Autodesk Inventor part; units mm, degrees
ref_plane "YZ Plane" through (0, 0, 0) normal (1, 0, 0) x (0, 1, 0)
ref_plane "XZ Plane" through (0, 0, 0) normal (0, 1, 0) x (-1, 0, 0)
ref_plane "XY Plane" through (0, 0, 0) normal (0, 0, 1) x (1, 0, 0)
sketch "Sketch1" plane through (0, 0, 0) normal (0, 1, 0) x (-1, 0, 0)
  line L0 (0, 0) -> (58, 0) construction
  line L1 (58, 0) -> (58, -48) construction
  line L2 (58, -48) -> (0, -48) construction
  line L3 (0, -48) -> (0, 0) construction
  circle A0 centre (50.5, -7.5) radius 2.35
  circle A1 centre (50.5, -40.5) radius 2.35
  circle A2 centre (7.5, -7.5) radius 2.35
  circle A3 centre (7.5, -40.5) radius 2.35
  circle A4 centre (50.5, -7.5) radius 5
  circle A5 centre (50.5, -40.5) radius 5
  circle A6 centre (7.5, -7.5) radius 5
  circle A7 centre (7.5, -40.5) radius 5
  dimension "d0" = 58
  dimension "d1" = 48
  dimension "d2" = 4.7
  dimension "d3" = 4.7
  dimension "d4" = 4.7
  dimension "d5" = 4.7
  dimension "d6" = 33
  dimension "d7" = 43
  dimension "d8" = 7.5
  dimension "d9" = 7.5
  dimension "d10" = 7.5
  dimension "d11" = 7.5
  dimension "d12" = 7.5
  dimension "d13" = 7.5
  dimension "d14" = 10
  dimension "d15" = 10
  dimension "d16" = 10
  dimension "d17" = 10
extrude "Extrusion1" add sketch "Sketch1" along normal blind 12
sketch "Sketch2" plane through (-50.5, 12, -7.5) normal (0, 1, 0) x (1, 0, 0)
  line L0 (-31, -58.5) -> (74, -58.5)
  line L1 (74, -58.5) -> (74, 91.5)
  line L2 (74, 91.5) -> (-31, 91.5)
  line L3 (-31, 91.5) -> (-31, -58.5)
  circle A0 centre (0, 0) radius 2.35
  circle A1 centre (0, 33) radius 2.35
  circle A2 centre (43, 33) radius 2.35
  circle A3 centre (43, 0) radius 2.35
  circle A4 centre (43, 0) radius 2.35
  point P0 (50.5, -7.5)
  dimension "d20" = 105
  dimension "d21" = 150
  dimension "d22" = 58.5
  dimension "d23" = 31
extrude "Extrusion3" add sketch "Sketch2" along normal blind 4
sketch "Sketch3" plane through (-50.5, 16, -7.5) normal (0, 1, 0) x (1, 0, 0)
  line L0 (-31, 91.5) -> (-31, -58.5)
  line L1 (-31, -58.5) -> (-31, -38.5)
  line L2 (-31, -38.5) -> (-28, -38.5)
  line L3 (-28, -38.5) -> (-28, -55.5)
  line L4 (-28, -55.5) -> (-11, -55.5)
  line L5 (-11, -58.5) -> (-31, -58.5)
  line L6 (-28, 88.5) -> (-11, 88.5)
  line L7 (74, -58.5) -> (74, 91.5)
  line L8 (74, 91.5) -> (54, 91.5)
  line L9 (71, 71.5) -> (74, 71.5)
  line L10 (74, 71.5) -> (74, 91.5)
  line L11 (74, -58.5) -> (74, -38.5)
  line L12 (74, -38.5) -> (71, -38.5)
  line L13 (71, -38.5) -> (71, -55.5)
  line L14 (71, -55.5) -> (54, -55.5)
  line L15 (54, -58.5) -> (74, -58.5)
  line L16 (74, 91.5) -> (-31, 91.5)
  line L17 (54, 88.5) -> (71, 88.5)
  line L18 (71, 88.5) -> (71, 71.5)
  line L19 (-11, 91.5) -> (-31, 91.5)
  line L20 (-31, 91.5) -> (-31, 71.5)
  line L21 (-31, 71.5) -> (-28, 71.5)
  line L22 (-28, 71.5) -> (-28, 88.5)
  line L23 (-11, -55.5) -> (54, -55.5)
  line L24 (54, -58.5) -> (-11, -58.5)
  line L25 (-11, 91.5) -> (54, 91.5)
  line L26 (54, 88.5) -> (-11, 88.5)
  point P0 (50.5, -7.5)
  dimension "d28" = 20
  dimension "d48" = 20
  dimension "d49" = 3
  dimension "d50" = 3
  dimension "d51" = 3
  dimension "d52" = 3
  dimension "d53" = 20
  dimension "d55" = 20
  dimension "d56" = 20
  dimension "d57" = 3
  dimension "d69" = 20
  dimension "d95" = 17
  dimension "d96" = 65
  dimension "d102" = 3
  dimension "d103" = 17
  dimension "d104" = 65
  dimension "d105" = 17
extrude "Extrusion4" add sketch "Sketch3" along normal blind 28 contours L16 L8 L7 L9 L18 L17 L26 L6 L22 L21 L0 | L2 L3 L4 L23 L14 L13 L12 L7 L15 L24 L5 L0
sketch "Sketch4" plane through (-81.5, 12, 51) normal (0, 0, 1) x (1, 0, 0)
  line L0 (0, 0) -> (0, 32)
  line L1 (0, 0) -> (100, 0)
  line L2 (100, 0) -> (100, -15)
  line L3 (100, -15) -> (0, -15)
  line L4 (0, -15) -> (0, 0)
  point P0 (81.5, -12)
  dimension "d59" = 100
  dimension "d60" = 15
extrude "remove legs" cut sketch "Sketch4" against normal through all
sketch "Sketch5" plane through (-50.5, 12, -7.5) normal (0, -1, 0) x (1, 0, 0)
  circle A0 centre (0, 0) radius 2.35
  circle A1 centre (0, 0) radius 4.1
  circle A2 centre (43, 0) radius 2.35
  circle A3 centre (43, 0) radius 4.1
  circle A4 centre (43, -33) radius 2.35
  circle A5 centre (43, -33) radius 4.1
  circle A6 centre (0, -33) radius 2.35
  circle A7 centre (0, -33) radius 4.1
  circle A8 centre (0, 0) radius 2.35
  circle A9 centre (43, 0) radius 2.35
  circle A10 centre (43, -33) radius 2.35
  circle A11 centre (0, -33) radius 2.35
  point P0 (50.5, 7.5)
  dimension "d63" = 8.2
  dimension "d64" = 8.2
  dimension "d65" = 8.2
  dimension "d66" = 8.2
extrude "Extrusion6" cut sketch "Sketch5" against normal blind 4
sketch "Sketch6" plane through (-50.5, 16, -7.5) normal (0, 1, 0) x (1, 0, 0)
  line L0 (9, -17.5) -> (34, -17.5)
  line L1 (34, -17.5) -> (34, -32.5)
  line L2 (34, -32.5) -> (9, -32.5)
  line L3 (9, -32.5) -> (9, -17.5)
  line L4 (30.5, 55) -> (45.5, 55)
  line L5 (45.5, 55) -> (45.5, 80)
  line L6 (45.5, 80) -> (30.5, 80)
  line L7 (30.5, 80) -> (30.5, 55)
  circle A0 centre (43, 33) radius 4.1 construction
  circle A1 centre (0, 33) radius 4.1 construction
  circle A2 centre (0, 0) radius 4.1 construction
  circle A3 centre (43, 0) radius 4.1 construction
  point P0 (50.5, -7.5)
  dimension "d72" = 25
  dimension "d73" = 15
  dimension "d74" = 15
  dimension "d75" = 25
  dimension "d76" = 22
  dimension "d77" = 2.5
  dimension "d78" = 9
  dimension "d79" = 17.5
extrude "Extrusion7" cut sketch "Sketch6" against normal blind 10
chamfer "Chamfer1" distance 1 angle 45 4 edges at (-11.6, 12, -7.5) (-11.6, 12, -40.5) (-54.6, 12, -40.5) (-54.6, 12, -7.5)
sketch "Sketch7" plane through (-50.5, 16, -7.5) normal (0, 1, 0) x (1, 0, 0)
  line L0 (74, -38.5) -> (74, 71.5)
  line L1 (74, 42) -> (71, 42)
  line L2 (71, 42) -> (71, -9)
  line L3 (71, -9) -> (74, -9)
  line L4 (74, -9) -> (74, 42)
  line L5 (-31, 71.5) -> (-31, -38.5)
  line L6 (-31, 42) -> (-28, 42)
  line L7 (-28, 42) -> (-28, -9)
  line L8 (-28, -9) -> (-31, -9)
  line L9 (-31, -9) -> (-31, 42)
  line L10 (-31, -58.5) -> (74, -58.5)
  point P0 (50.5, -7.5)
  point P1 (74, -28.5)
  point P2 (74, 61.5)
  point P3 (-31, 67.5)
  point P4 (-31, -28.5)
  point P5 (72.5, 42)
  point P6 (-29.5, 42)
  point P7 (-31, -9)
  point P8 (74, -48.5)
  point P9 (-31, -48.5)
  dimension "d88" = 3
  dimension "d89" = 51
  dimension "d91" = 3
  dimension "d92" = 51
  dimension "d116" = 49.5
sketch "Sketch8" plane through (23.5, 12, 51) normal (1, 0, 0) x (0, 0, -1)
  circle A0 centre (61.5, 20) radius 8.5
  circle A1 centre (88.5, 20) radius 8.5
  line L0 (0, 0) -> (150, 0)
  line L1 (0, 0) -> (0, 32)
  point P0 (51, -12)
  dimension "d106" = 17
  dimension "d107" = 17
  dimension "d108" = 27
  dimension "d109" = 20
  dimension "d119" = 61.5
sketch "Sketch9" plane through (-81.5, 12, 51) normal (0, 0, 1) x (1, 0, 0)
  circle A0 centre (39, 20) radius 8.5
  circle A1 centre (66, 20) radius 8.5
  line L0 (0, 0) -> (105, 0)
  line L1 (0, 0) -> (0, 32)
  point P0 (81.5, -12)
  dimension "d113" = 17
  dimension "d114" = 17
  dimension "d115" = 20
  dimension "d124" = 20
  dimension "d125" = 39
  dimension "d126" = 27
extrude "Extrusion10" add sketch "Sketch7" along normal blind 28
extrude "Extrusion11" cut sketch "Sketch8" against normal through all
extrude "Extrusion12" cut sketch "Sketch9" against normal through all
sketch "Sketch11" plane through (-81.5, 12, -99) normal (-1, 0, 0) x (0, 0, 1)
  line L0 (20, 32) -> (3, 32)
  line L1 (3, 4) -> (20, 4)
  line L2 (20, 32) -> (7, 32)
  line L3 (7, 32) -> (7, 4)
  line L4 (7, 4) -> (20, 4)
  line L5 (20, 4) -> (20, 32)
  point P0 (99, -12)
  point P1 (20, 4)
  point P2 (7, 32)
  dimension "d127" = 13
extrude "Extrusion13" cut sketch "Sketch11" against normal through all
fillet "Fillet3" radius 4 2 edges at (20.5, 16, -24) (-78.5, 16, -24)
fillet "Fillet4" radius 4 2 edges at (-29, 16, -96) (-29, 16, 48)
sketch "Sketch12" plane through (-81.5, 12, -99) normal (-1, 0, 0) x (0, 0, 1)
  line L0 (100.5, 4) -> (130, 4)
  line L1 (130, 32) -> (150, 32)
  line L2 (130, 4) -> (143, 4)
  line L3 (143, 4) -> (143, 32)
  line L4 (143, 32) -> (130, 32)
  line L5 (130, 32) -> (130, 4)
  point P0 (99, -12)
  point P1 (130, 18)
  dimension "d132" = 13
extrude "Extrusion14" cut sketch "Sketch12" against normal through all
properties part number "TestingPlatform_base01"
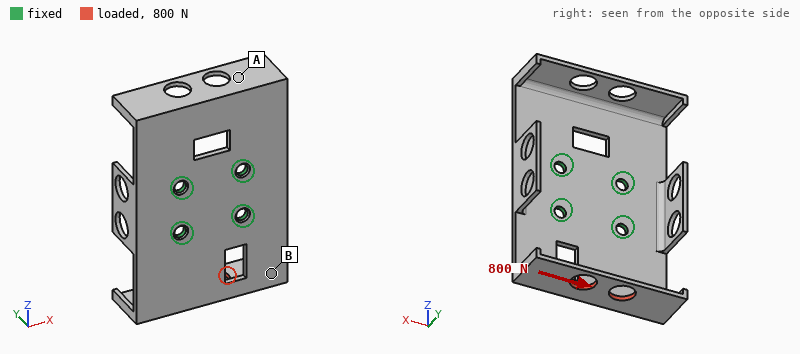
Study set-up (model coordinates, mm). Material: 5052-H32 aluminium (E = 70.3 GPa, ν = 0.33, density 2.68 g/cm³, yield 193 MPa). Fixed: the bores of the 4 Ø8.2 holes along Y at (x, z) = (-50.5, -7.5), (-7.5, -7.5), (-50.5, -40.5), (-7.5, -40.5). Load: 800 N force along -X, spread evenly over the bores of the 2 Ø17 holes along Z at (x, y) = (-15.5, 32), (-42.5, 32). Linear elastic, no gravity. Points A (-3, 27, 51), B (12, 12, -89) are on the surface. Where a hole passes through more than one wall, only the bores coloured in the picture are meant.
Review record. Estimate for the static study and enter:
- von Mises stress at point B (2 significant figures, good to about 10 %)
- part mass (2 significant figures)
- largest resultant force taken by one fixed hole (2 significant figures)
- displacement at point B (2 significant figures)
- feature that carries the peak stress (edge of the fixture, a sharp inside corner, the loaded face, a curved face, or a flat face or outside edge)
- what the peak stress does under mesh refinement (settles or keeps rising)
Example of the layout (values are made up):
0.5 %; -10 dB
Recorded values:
23 MPa; 220 g; 780 N; 0.28 mm; edge of the fixture; keeps rising
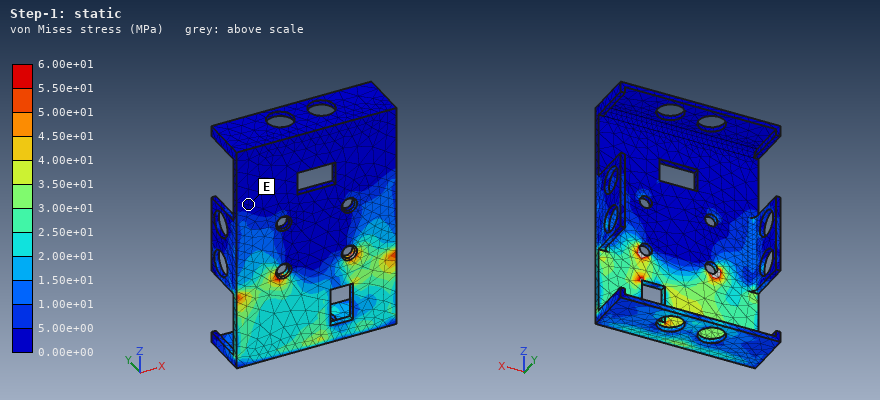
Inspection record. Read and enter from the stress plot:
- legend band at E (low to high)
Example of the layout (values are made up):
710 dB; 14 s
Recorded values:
0.00e+00 to 5.00e+00 MPa
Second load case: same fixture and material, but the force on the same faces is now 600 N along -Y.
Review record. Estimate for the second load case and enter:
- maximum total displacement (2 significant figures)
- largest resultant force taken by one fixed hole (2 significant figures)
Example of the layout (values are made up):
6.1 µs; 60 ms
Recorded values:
1.2 mm; 520 N
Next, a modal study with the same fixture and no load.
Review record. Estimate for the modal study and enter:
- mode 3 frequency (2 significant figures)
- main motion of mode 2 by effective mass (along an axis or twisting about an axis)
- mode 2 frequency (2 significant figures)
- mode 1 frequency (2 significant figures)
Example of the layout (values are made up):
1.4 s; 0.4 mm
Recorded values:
890 Hz; along Y; 620 Hz; 580 Hz
